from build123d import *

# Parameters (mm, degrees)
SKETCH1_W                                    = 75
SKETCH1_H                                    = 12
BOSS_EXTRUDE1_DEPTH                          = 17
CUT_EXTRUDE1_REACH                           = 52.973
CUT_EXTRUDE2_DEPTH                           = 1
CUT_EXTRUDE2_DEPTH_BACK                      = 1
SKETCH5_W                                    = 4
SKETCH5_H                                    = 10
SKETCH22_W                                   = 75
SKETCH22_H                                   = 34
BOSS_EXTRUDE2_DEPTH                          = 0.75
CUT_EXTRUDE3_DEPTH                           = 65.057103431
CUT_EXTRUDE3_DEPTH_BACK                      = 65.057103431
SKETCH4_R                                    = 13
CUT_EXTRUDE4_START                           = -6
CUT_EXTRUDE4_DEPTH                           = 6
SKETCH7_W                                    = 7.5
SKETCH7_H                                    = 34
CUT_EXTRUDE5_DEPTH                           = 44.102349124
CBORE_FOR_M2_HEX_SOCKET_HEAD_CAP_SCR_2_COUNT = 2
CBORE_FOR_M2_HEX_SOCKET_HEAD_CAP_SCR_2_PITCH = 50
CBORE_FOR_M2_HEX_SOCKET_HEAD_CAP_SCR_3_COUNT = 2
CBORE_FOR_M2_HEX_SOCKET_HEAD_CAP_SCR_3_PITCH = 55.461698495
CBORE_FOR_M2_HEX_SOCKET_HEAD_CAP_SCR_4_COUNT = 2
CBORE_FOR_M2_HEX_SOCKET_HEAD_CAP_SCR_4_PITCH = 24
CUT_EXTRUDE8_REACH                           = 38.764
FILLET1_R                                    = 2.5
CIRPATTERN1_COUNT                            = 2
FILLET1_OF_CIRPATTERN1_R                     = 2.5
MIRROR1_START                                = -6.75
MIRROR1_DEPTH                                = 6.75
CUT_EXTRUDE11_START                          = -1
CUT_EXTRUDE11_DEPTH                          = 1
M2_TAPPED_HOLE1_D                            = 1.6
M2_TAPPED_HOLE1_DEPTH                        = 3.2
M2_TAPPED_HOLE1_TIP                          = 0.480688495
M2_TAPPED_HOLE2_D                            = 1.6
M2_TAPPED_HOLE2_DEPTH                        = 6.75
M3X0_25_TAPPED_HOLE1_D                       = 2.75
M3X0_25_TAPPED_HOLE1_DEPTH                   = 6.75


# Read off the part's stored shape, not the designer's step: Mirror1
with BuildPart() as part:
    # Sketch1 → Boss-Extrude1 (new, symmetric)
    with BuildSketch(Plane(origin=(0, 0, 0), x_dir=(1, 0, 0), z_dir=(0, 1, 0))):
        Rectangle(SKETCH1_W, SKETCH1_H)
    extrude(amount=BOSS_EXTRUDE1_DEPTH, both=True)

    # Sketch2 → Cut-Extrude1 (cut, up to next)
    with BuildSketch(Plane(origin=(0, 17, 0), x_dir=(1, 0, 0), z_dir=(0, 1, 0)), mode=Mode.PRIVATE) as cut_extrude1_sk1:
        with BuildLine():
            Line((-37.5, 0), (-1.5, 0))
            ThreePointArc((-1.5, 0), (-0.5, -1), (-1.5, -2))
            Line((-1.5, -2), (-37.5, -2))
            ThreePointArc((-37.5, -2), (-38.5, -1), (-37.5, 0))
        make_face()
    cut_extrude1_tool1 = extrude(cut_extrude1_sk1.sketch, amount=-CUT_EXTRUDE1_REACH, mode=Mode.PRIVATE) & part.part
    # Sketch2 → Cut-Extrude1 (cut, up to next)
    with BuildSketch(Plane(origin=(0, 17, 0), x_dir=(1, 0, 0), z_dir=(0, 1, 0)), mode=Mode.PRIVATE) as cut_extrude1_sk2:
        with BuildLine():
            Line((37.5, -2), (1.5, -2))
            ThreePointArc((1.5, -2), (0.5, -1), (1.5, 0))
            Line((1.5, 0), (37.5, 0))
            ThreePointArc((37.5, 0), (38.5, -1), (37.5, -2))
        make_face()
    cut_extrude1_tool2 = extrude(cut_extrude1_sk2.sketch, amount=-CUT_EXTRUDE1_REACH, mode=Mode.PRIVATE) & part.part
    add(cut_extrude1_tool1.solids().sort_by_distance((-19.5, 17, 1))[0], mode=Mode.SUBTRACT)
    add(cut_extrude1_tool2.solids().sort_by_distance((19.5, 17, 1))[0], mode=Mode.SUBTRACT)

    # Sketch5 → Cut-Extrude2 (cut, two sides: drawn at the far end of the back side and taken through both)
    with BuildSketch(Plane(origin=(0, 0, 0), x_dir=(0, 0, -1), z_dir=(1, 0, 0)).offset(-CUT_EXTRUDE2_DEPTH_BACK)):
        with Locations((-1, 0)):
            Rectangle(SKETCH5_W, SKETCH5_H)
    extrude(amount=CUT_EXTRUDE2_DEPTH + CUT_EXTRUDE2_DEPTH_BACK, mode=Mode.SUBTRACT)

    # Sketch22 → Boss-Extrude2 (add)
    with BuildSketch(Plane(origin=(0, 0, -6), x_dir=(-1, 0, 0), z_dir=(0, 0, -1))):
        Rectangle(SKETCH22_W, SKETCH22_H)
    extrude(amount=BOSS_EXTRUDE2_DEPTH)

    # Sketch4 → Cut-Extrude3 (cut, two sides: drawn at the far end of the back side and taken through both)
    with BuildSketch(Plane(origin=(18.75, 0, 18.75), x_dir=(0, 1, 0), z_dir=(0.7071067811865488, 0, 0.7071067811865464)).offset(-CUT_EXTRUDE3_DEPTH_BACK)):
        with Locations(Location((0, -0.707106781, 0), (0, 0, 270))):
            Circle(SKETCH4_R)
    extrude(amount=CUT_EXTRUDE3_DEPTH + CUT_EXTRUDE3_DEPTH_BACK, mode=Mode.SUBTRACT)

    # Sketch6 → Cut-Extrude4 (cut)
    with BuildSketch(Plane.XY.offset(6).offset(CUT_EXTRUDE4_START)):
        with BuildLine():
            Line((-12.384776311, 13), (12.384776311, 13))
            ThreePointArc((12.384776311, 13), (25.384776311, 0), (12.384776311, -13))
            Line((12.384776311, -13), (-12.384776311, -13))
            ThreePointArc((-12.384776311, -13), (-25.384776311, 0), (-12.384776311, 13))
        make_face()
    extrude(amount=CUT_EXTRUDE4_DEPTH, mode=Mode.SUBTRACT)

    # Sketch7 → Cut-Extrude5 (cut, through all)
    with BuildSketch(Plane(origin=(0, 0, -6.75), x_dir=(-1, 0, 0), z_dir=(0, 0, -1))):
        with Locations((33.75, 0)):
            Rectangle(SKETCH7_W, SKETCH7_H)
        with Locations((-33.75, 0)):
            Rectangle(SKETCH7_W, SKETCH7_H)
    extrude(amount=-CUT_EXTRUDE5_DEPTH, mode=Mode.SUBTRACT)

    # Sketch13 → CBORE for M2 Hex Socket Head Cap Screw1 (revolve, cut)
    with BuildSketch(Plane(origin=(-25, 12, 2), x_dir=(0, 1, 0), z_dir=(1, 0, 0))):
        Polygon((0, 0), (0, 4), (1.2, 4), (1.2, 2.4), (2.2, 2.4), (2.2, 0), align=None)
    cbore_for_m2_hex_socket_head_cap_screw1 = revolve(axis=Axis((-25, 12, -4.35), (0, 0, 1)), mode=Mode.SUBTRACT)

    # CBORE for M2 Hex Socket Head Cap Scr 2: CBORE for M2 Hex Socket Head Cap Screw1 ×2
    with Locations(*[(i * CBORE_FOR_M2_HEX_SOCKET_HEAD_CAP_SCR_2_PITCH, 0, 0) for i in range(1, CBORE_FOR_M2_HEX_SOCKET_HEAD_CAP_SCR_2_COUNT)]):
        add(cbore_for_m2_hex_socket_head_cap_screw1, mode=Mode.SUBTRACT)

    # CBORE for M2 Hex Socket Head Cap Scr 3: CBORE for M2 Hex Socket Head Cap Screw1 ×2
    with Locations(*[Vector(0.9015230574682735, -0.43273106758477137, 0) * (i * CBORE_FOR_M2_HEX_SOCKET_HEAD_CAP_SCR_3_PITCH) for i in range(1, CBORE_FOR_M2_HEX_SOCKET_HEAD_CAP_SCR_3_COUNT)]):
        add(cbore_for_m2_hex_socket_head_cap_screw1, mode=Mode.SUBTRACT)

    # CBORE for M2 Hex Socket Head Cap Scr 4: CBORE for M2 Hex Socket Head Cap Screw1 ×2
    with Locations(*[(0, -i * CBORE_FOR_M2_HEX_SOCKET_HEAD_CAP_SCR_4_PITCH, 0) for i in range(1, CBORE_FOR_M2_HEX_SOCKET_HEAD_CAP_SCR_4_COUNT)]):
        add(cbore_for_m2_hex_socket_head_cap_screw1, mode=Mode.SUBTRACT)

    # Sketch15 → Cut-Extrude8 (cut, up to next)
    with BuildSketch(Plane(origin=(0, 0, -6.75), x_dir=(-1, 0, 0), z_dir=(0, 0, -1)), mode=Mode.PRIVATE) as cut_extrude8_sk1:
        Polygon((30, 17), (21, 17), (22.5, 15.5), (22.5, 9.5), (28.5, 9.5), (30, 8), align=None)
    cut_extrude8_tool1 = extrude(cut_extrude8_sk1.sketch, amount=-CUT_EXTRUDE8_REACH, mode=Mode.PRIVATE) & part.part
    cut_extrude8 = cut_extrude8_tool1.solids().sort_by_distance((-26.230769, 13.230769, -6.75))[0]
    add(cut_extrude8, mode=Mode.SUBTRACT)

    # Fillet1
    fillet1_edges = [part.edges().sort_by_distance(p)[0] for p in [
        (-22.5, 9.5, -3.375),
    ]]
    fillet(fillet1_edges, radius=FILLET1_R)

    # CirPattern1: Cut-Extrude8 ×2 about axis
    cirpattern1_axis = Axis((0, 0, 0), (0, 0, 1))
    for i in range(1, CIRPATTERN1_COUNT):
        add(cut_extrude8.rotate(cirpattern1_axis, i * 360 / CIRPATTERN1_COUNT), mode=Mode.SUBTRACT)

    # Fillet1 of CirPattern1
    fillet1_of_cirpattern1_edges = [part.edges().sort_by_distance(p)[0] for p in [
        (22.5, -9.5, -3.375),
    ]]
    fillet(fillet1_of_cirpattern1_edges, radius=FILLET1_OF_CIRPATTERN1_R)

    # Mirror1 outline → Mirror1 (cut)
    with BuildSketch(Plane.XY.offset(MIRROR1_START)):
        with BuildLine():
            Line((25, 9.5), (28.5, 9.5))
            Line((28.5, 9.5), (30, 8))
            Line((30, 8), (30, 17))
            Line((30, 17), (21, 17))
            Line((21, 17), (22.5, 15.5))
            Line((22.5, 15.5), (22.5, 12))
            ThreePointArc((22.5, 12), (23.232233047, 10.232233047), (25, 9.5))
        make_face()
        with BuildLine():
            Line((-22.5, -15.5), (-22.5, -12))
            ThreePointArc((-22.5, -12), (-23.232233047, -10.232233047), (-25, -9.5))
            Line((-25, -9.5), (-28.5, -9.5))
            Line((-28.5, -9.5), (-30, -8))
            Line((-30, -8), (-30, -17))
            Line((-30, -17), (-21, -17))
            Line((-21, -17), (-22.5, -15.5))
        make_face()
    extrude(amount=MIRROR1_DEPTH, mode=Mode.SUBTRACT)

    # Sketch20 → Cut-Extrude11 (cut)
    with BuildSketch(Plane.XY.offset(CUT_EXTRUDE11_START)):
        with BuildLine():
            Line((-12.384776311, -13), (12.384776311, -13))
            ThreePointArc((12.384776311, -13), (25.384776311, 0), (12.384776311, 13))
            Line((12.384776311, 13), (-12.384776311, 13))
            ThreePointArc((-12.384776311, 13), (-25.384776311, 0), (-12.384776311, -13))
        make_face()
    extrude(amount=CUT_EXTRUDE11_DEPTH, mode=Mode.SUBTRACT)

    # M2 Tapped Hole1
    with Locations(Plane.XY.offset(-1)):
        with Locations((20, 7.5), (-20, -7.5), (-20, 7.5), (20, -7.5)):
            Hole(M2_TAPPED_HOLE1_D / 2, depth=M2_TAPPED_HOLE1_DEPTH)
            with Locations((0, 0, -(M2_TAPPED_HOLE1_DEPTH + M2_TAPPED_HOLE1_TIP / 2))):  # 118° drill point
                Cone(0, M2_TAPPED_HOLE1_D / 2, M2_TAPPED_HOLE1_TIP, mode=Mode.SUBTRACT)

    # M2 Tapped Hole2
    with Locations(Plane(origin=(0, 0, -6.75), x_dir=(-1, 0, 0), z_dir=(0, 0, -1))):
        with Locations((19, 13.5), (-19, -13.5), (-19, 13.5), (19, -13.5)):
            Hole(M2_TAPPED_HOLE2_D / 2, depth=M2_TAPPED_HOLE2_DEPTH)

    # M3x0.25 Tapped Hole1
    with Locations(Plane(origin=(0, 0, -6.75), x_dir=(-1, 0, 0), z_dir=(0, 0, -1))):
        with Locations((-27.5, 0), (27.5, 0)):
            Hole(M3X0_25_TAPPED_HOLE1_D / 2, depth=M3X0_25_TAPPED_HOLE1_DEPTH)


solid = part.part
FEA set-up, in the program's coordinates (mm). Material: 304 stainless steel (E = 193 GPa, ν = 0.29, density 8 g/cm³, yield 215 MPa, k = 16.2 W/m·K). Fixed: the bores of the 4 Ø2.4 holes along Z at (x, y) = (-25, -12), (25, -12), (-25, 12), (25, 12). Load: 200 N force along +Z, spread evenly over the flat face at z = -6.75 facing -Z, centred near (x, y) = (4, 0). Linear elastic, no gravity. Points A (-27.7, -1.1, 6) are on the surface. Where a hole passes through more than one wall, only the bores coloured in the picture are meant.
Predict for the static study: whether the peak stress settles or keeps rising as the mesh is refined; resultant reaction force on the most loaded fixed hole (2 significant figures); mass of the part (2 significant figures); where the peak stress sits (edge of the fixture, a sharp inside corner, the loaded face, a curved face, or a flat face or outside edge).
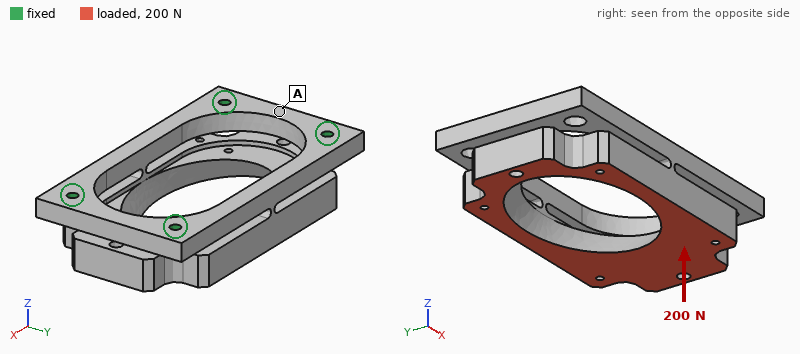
keeps rising
91 N
79 g
a sharp inside corner
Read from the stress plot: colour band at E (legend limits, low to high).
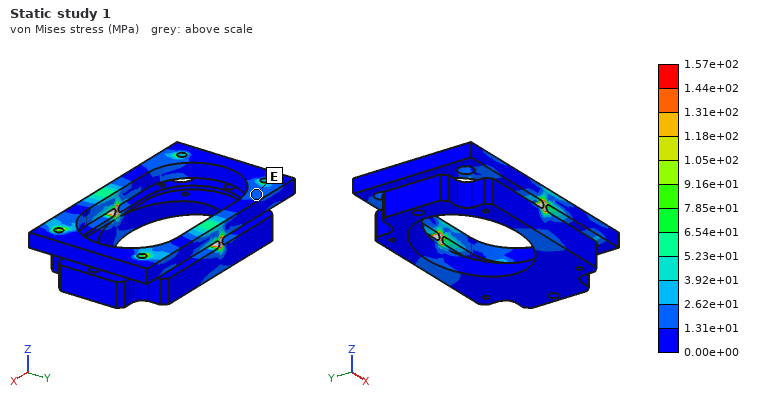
1.31e+01 to 2.62e+01 MPa
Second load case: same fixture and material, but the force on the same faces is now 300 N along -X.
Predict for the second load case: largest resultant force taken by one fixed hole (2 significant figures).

90 N
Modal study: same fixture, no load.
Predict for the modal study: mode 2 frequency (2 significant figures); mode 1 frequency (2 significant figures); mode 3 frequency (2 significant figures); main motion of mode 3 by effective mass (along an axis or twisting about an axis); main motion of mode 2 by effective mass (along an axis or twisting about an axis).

1900 Hz
340 Hz
2100 Hz
along Y
along Z
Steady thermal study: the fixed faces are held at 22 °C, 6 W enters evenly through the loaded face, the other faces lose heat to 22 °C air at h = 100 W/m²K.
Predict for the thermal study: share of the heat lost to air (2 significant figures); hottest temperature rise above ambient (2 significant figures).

98 %
24 K
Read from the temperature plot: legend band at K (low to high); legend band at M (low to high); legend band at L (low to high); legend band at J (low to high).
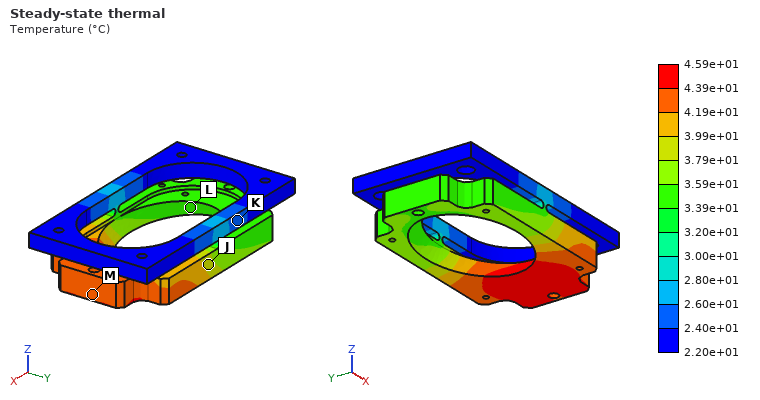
2.40e+01 to 2.60e+01 °C
4.19e+01 to 4.39e+01 °C
3.39e+01 to 3.59e+01 °C
3.79e+01 to 3.99e+01 °C
